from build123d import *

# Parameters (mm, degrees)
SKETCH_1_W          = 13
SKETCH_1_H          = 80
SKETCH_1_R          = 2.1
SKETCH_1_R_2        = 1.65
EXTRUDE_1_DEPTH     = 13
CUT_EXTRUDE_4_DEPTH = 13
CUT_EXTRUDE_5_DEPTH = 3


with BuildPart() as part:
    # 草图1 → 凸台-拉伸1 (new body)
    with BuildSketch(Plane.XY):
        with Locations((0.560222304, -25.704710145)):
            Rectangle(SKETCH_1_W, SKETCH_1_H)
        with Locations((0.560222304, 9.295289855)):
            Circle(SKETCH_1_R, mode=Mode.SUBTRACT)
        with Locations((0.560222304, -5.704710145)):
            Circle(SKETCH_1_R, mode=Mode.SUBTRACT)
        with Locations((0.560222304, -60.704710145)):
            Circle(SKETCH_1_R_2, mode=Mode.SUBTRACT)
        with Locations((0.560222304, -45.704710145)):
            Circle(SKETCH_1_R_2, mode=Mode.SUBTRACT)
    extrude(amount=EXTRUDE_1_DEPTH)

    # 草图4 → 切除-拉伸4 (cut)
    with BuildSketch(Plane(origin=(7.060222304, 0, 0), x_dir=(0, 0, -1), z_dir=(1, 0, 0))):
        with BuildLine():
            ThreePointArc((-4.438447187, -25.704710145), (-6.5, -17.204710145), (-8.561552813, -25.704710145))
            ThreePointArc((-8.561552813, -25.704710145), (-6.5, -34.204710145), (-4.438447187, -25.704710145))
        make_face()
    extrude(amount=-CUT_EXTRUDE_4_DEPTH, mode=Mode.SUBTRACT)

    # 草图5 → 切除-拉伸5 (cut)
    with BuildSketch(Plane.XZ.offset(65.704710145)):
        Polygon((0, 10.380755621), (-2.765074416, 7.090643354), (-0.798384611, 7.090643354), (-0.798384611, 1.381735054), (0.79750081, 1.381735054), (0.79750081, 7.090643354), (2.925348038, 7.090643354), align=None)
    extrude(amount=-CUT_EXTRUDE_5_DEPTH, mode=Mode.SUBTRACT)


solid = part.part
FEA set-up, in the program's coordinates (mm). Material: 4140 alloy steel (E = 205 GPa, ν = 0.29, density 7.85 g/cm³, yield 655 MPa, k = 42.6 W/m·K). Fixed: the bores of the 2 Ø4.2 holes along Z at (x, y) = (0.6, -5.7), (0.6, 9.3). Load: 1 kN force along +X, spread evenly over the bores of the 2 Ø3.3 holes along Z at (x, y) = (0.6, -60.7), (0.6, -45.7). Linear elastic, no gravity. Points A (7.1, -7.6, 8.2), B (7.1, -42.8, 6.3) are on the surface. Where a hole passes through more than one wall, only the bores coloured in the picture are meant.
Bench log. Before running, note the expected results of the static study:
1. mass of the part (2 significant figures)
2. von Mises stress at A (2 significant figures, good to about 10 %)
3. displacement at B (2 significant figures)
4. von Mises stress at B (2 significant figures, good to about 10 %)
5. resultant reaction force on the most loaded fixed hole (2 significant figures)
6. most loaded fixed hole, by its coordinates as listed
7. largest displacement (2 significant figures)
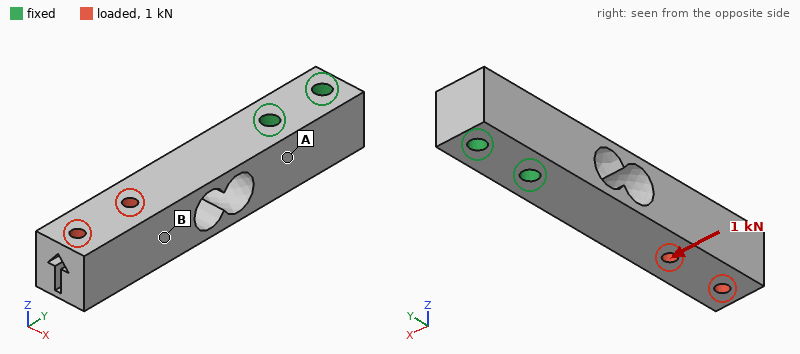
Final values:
88 g
100 MPa
0.11 mm
26 MPa
2.5 kN
(0.6, -5.7)
0.22 mm
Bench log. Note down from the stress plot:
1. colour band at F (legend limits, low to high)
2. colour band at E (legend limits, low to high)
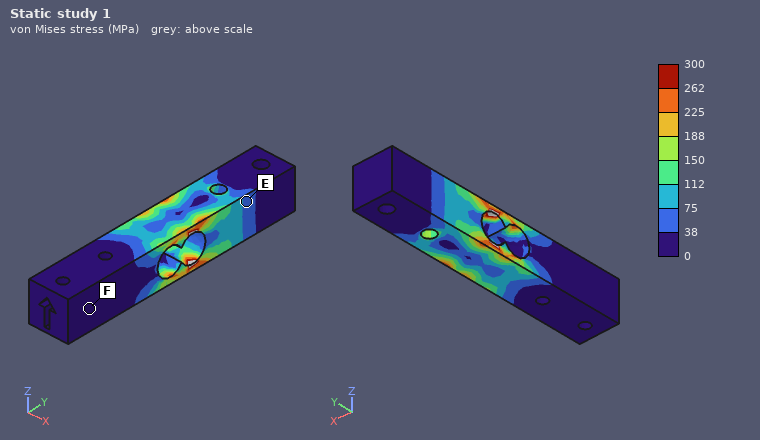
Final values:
0 to 38 MPa
38 to 75 MPa
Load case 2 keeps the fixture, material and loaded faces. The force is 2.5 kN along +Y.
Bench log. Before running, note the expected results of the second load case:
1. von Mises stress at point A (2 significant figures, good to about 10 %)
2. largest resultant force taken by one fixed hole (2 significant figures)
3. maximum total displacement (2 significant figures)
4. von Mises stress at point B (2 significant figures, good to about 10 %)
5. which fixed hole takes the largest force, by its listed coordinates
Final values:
6.2 MPa
2.3 kN
7.4 µm
8.8 MPa
(0.6, -5.7)
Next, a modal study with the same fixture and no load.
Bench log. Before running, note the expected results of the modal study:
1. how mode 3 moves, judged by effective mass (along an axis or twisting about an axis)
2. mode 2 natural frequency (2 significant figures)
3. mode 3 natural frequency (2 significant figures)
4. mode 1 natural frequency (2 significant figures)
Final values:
twisting about Y
2100 Hz
7800 Hz
2100 Hz
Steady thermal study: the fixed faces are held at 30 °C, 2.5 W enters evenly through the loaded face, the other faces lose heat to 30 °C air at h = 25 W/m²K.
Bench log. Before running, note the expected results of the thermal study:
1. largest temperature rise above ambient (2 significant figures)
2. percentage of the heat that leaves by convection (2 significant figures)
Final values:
18 K
40 %
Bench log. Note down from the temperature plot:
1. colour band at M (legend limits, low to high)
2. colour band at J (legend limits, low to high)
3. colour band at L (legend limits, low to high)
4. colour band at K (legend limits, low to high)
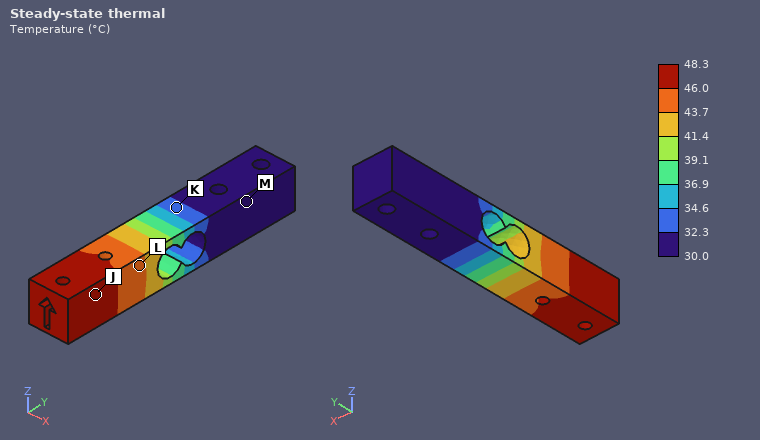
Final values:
30.0 to 32.3 °C
46.0 to 48.3 °C
43.7 to 46.0 °C
32.3 to 34.6 °C
